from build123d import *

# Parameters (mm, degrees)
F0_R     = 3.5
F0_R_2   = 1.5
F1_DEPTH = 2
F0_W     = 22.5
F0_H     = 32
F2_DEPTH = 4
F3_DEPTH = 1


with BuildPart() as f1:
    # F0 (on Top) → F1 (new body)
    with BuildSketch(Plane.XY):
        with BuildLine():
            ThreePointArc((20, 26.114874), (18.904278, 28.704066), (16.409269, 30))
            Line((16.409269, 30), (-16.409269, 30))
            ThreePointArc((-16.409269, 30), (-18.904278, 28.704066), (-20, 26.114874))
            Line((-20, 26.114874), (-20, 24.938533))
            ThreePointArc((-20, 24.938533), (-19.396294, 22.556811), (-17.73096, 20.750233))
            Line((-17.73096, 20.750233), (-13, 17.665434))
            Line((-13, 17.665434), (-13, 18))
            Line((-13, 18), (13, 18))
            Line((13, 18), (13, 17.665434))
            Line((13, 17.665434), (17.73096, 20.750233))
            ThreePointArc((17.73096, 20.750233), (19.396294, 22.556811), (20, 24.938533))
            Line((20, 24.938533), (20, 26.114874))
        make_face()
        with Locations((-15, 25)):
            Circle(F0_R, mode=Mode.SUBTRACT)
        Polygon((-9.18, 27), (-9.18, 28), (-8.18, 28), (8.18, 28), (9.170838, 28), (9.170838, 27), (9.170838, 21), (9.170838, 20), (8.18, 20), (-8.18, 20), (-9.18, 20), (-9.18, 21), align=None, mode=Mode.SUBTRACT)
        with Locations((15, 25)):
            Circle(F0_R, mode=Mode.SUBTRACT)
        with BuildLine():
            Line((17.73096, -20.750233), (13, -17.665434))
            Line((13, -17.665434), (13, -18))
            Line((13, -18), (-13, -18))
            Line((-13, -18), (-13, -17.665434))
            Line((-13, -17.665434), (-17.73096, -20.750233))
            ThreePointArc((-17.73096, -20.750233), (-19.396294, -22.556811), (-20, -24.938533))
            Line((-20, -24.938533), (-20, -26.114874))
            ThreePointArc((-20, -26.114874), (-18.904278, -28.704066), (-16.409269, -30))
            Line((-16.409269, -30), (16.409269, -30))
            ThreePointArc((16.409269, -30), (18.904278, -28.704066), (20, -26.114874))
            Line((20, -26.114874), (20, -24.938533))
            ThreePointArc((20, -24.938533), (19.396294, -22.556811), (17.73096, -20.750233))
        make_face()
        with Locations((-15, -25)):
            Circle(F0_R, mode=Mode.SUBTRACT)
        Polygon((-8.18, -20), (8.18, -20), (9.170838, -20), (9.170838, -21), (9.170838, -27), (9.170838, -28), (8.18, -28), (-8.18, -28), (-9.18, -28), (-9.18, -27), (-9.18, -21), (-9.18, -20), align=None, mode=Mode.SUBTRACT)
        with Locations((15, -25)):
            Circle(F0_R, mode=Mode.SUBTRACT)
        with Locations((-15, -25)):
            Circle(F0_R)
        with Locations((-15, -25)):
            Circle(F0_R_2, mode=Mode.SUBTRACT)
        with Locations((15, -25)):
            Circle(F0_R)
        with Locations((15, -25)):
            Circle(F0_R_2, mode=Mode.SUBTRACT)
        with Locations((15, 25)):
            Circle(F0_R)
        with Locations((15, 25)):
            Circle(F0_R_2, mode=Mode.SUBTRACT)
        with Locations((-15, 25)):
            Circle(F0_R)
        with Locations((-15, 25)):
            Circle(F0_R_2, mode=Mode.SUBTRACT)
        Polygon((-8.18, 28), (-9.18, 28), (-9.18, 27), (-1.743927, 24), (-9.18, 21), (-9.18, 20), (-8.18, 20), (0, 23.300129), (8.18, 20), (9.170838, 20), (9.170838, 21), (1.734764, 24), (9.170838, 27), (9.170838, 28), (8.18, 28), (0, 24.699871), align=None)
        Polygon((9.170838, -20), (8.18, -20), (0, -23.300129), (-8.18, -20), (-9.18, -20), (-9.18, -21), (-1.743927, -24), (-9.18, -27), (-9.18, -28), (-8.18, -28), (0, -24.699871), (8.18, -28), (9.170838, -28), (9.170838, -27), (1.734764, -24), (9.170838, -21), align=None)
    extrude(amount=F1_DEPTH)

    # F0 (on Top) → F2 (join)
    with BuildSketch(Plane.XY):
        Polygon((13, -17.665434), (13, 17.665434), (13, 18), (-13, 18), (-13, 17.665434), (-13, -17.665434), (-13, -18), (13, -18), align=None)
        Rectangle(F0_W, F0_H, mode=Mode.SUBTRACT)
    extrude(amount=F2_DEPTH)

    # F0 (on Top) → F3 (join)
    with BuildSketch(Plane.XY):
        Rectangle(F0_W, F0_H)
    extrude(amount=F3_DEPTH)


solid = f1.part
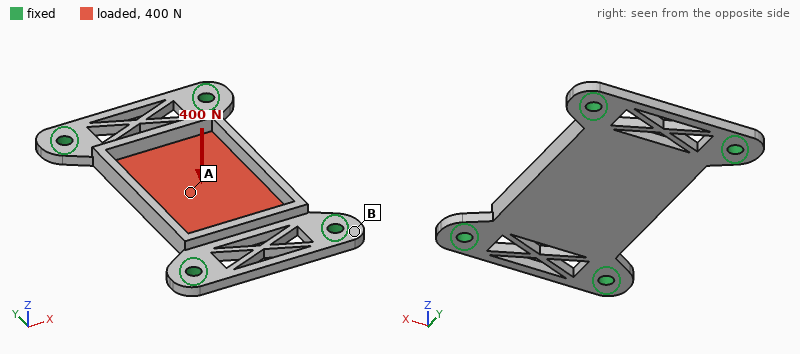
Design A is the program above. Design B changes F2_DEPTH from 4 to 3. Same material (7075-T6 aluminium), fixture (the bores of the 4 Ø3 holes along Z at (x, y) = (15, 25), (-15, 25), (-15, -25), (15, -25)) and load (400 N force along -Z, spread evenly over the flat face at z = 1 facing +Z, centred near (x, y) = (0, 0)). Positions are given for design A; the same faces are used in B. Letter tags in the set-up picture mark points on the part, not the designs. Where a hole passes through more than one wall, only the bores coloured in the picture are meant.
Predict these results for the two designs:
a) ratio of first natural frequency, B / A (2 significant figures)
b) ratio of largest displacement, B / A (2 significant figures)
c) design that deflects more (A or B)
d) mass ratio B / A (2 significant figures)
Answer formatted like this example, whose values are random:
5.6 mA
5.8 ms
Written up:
0.86
1.4
B
0.93
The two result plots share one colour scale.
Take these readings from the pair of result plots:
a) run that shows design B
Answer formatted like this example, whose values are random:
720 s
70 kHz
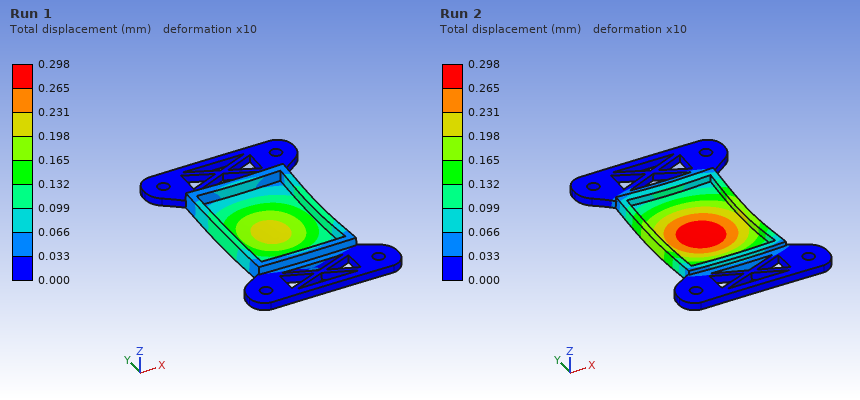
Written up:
Run 2
